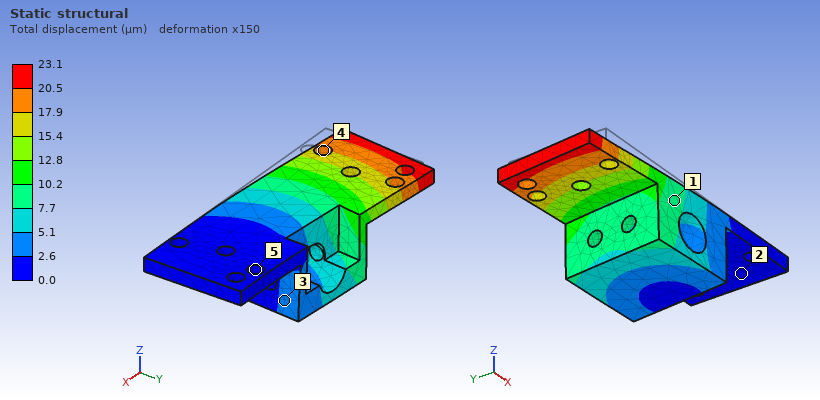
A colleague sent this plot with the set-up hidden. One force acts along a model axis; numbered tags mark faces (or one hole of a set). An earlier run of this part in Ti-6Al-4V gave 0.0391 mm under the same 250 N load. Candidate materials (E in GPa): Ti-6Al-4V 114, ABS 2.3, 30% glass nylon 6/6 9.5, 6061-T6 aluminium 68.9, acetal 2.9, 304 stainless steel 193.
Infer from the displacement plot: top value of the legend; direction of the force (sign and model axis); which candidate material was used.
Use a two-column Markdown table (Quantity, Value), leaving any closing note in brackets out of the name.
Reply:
| Quantity | Value |
|---|---|
| top value of the legend | 23.1 µm |
| direction of the force | +Y |
| which candidate material was used | 304 stainless steel |
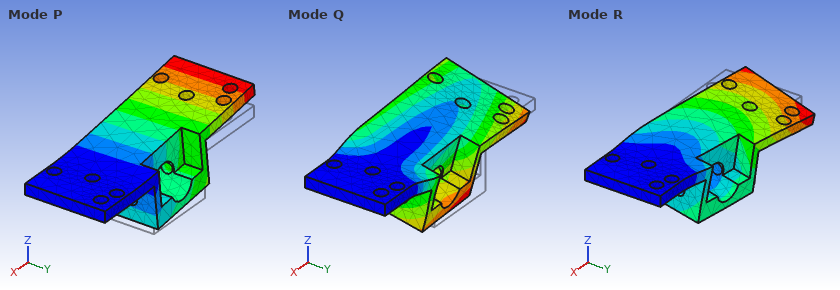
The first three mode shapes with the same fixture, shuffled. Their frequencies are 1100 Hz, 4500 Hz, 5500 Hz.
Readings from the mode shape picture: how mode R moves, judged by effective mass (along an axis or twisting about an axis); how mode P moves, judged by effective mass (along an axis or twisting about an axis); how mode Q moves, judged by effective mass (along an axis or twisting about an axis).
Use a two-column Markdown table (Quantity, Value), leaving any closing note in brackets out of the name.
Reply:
| Quantity | Value |
|---|---|
| how mode R moves, judged by effective mass | along Y |
| how mode P moves, judged by effective mass | along Z |
| how mode Q moves, judged by effective mass | along Y |
